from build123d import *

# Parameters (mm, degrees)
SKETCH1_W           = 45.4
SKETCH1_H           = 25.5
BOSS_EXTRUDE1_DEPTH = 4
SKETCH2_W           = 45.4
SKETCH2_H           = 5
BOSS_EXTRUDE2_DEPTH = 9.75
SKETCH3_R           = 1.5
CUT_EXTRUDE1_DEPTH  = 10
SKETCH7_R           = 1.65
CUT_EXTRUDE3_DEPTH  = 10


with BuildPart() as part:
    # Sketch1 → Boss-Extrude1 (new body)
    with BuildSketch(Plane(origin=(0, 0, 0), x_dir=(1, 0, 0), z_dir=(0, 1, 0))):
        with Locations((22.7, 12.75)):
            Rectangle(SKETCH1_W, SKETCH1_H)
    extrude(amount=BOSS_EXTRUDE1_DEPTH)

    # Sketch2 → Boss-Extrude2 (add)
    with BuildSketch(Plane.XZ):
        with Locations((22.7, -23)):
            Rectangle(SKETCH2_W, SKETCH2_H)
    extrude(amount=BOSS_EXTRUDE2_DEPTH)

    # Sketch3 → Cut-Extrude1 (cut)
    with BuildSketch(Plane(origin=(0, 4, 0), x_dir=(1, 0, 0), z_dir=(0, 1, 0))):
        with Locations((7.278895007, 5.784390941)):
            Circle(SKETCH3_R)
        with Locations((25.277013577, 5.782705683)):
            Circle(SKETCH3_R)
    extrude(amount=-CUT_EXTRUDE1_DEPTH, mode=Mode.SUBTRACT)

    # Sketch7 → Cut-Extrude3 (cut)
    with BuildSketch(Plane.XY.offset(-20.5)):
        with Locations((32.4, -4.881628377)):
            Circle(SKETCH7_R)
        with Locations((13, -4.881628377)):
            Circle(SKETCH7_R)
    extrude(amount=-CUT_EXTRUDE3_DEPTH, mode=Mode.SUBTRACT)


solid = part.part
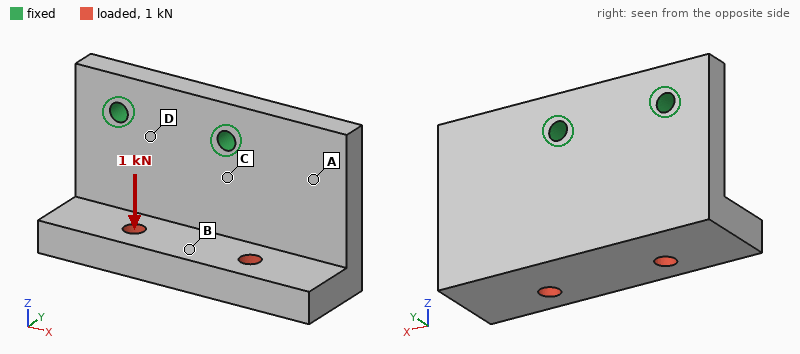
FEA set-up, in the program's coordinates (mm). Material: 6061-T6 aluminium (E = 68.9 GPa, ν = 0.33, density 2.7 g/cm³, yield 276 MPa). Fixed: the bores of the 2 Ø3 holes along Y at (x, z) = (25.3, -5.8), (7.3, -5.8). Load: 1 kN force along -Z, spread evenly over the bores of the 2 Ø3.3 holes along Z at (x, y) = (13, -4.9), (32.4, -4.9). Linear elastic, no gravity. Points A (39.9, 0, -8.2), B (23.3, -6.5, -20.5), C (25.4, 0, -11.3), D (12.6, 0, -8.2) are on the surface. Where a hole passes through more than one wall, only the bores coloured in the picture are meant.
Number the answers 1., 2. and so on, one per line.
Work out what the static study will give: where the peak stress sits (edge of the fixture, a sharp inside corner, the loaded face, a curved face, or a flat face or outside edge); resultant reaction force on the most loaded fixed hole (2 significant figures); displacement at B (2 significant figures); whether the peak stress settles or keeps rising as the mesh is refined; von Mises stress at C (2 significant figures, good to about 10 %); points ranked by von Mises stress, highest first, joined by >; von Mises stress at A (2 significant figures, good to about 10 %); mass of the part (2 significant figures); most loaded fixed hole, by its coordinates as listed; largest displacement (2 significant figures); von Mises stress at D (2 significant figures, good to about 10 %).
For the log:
1. edge of the fixture
2. 820 N
3. 0.090 mm
4. keeps rising
5. 83 MPa
6. C > D > A > B
7. 31 MPa
8. 18 g
9. (25.3, -5.8)
10. 0.14 mm
11. 48 MPa
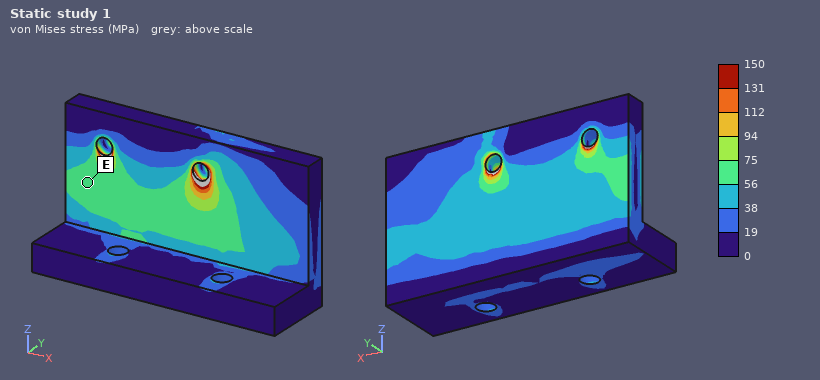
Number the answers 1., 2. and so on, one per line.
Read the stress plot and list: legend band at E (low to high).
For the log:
1. 56 to 75 MPa
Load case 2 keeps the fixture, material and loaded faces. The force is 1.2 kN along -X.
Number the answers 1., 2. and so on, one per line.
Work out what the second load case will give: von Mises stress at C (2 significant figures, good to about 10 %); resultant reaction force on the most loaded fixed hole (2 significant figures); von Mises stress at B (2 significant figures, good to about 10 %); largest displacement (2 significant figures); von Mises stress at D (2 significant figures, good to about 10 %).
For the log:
1. 52 MPa
2. 1.2 kN
3. 23 MPa
4. 0.10 mm
5. 42 MPa
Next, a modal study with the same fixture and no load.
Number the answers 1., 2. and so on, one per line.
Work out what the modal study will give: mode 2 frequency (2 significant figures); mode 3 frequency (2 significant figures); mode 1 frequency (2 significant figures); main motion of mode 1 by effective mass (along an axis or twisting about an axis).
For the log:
1. 5700 Hz
2. 11 kHz
3. 3700 Hz
4. along Y
